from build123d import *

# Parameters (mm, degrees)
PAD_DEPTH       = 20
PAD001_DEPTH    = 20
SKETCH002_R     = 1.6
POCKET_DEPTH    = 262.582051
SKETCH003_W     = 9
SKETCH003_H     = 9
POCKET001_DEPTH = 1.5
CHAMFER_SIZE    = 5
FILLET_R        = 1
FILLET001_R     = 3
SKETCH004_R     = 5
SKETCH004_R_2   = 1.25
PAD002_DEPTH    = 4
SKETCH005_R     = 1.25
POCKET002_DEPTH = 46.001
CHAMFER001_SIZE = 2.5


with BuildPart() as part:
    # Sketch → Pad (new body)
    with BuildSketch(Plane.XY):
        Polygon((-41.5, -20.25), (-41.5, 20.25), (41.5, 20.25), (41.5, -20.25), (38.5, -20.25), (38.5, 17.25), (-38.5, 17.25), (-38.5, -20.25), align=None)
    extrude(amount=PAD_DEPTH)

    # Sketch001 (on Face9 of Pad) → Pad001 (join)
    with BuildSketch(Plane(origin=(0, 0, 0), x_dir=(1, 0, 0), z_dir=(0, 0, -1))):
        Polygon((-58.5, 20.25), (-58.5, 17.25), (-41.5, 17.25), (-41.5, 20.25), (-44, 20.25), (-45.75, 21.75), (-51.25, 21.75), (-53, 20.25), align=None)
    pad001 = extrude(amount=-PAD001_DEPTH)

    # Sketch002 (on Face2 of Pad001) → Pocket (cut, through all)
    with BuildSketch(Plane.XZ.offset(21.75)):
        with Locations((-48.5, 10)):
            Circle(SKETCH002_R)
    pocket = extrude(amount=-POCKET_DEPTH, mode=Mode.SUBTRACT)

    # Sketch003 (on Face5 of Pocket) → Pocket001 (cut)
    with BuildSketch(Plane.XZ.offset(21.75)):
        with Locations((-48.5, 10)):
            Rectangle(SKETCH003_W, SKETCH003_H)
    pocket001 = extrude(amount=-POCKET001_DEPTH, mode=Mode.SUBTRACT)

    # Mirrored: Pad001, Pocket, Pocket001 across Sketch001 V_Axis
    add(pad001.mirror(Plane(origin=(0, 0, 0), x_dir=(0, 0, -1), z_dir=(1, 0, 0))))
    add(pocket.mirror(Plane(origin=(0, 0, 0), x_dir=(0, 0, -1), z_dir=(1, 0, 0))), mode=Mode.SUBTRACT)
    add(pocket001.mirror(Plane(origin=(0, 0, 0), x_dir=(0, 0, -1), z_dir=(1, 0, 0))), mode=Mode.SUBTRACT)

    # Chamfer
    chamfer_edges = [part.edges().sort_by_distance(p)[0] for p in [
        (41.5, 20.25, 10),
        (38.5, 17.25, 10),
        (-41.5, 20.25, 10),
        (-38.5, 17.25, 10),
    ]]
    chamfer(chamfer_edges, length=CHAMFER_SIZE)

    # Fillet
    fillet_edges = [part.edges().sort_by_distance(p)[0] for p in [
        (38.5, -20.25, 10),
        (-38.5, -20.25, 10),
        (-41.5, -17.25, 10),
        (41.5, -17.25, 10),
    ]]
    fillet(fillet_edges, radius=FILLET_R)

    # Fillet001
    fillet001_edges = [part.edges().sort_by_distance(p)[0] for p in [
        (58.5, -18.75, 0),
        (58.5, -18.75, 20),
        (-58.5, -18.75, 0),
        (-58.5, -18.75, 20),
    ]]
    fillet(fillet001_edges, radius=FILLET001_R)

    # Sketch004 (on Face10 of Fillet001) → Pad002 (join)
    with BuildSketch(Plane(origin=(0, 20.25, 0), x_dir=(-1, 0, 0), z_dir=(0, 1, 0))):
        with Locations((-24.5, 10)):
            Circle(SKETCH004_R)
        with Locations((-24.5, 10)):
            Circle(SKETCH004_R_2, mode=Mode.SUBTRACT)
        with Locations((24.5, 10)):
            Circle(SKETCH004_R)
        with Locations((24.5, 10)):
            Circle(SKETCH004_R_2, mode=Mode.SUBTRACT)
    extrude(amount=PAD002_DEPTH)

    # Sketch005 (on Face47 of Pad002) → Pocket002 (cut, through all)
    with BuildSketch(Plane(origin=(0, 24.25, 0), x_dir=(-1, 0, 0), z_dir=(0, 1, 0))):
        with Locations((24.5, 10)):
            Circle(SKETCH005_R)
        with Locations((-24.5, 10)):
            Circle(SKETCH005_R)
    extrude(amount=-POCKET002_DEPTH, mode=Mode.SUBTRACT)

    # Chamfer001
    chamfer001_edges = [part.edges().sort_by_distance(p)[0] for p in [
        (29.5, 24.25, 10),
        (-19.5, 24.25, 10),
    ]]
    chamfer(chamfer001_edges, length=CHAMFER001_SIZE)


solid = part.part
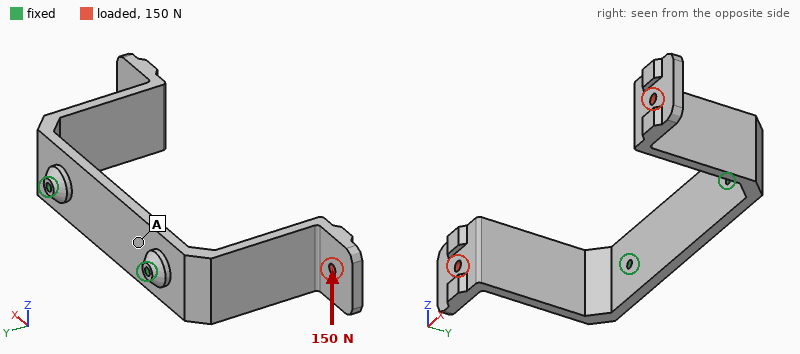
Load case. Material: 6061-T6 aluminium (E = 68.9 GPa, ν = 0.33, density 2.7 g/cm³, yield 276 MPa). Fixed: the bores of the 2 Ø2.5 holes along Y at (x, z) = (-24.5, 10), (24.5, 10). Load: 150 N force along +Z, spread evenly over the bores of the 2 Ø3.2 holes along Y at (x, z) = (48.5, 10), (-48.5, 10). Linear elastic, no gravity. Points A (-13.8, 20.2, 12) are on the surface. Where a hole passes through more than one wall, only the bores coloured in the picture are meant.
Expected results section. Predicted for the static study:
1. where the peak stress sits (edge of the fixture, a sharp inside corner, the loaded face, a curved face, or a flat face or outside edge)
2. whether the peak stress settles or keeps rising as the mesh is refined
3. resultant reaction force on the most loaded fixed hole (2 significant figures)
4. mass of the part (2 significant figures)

edge of the fixture
keeps rising
75 N
33 g
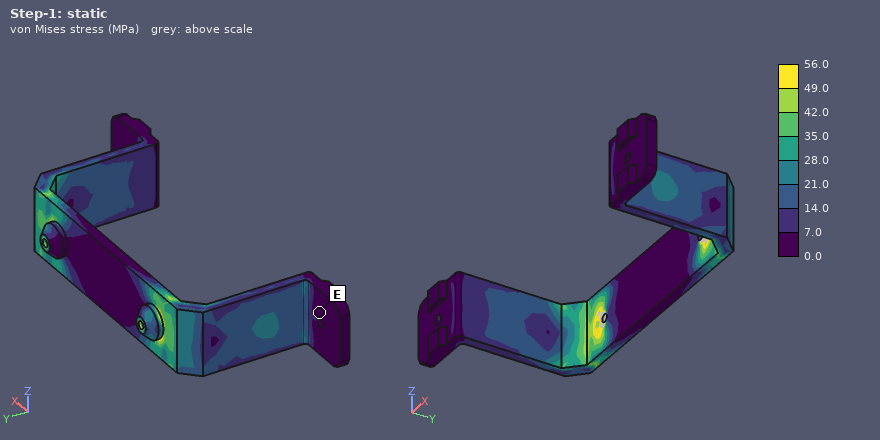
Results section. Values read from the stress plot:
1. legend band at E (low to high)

0.0 to 7.0 MPa
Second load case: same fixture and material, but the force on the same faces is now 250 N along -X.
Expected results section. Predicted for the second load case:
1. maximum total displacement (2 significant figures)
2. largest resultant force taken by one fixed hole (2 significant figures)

1.3 mm
130 N
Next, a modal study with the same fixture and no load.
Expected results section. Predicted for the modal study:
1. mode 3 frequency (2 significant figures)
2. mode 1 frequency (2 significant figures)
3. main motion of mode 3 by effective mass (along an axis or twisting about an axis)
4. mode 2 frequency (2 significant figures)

1400 Hz
750 Hz
along Z
750 Hz
